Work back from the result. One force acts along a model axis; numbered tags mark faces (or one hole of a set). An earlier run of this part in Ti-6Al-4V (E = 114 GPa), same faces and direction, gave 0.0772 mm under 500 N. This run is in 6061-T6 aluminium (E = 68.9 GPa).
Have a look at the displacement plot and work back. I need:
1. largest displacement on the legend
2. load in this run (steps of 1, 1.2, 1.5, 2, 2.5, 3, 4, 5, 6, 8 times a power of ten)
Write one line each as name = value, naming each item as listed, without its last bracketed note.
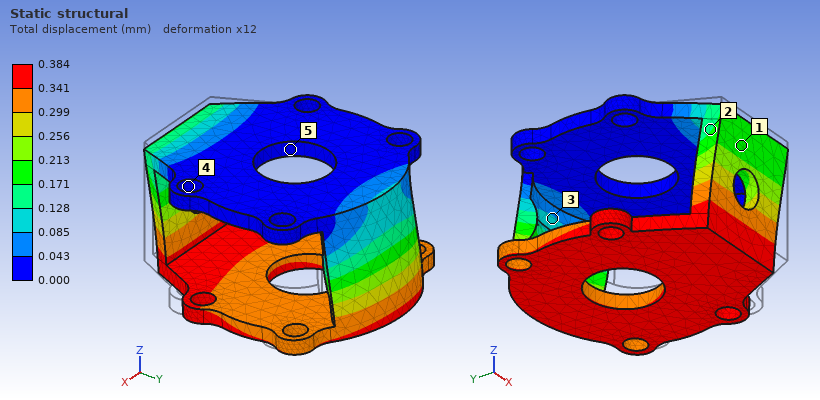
largest displacement on the legend = 0.384 mm
load in this run = 1.5 kN
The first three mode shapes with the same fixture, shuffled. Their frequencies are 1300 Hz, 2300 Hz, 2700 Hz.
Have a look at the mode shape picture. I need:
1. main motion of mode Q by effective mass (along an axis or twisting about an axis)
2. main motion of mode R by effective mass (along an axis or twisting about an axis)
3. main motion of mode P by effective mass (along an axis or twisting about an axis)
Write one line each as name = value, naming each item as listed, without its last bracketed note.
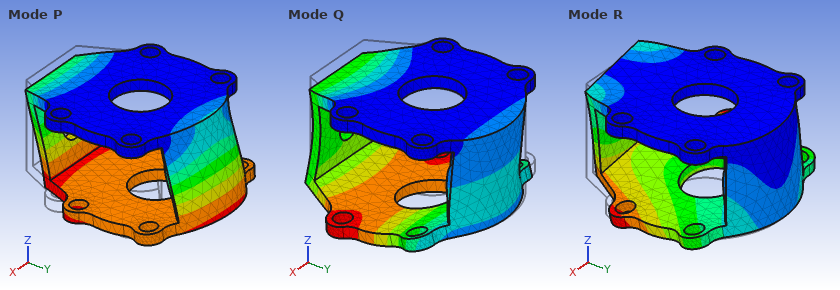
main motion of mode Q by effective mass = along Z
main motion of mode R by effective mass = along X
main motion of mode P by effective mass = along Y
